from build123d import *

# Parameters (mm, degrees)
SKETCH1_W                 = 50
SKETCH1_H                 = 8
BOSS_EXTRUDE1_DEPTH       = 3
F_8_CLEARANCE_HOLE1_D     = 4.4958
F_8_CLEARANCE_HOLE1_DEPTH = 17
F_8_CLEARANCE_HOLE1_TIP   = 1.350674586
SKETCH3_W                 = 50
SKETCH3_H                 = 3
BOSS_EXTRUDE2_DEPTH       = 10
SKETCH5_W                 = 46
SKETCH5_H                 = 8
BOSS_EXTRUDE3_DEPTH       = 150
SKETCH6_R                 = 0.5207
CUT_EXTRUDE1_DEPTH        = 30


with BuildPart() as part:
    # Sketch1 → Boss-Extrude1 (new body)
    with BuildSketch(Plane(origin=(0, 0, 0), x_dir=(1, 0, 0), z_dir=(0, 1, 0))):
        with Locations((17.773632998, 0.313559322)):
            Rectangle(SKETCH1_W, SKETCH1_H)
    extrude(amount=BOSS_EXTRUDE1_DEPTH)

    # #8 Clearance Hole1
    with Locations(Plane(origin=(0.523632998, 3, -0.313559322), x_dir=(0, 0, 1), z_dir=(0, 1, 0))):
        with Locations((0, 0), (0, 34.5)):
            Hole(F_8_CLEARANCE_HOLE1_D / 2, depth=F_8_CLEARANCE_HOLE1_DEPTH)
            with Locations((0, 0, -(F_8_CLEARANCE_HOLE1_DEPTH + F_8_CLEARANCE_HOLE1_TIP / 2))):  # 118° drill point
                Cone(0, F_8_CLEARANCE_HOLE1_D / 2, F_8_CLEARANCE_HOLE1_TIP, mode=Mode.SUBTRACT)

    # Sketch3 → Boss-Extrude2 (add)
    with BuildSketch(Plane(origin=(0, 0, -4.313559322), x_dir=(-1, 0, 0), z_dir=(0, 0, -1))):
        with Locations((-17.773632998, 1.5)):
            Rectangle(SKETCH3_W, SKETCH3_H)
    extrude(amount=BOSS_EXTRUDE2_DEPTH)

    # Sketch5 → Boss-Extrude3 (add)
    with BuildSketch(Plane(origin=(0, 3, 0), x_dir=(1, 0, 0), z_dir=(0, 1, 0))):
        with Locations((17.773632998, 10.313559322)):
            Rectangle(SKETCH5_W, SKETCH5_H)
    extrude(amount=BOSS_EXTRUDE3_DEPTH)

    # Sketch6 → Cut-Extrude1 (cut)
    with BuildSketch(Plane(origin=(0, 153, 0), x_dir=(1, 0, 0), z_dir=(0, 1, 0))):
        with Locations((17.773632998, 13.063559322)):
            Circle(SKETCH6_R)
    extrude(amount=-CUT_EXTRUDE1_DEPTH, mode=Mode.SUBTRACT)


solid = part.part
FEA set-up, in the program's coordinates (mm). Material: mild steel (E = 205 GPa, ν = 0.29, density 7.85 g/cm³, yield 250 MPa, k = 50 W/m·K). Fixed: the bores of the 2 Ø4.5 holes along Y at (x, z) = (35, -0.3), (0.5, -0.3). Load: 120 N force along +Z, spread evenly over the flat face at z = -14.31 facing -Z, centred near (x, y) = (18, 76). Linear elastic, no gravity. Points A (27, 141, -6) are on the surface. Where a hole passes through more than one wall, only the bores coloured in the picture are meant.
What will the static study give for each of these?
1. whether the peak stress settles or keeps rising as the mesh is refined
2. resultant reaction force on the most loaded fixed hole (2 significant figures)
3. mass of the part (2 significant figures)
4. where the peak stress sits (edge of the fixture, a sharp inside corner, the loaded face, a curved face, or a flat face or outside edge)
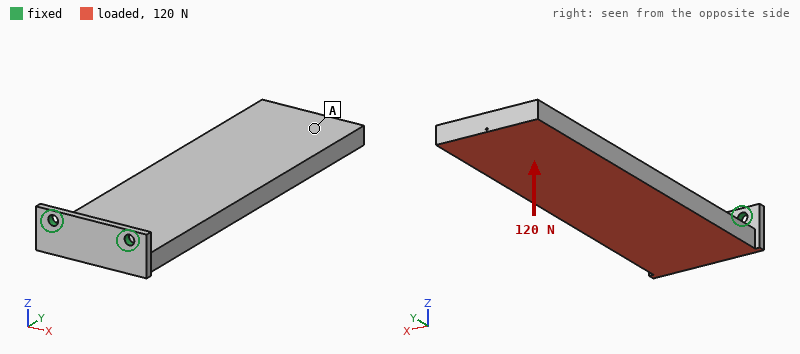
keeps rising
79 N
450 g
edge of the fixture
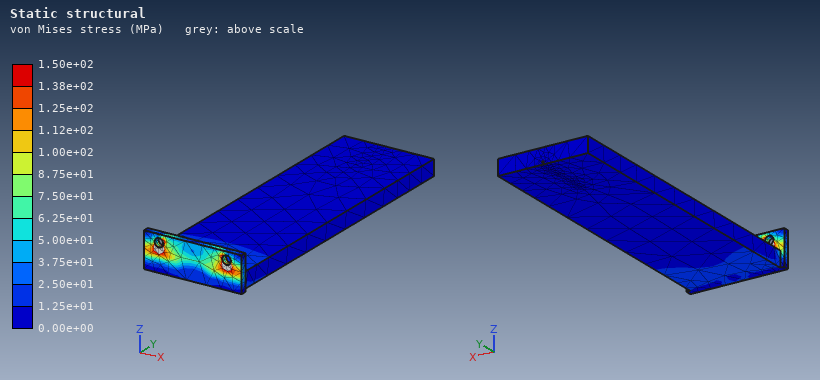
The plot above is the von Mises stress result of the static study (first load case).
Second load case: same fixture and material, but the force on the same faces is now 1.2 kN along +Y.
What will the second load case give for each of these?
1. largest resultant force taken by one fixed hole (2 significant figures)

600 N
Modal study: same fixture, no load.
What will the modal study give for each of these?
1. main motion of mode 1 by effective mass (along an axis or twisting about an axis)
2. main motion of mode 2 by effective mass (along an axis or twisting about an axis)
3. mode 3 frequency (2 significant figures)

along Z
along X
1300 Hz
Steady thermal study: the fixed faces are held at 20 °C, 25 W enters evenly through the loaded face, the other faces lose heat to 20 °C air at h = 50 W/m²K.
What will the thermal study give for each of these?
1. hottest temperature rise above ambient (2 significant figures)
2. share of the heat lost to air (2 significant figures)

39 K
66 %
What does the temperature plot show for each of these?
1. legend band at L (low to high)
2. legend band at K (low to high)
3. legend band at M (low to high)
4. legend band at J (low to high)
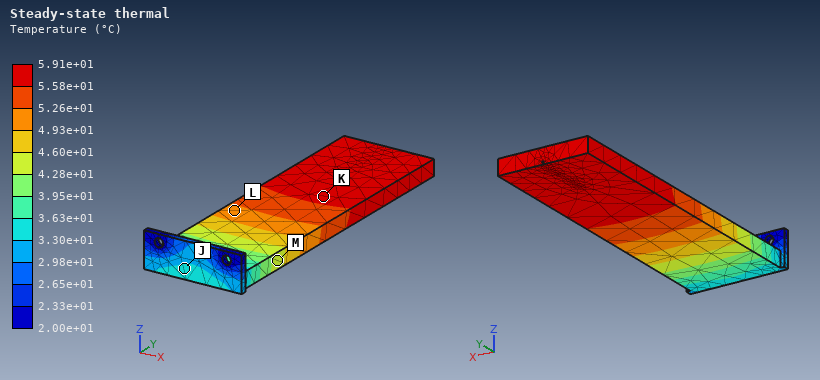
4.93e+01 to 5.26e+01 °C
5.58e+01 to 5.91e+01 °C
4.28e+01 to 4.60e+01 °C
3.30e+01 to 3.63e+01 °C
